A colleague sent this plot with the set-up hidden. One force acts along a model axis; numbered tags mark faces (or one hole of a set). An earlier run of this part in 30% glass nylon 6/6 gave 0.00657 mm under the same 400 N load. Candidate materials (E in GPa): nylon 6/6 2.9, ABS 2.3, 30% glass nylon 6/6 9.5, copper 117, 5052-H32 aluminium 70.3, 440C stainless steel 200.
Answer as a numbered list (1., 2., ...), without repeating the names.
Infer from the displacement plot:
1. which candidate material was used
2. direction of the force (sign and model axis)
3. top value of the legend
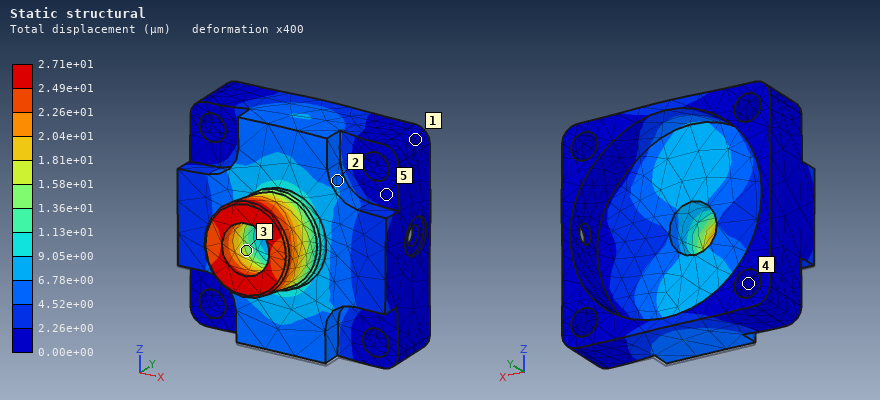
1. ABS
2. +Z
3. 2.71e+01 µm
